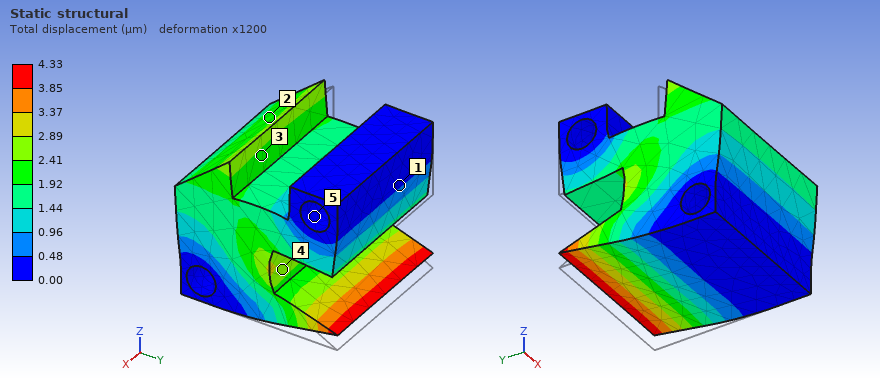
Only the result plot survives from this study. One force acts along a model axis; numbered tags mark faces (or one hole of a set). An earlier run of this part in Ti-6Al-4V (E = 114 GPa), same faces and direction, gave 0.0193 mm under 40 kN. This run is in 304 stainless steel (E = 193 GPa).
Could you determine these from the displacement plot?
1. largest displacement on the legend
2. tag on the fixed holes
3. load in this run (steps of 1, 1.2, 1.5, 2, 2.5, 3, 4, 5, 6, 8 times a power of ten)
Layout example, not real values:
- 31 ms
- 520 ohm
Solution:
- 4.33 µm
- 5
- 15 kN
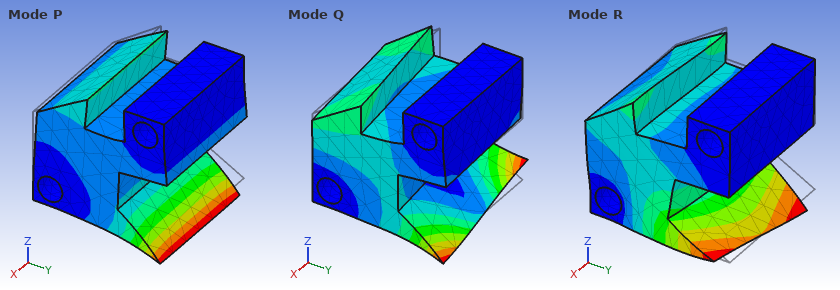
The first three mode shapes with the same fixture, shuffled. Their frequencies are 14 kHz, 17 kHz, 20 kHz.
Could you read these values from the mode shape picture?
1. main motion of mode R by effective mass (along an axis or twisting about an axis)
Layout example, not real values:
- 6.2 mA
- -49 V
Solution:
- along X
